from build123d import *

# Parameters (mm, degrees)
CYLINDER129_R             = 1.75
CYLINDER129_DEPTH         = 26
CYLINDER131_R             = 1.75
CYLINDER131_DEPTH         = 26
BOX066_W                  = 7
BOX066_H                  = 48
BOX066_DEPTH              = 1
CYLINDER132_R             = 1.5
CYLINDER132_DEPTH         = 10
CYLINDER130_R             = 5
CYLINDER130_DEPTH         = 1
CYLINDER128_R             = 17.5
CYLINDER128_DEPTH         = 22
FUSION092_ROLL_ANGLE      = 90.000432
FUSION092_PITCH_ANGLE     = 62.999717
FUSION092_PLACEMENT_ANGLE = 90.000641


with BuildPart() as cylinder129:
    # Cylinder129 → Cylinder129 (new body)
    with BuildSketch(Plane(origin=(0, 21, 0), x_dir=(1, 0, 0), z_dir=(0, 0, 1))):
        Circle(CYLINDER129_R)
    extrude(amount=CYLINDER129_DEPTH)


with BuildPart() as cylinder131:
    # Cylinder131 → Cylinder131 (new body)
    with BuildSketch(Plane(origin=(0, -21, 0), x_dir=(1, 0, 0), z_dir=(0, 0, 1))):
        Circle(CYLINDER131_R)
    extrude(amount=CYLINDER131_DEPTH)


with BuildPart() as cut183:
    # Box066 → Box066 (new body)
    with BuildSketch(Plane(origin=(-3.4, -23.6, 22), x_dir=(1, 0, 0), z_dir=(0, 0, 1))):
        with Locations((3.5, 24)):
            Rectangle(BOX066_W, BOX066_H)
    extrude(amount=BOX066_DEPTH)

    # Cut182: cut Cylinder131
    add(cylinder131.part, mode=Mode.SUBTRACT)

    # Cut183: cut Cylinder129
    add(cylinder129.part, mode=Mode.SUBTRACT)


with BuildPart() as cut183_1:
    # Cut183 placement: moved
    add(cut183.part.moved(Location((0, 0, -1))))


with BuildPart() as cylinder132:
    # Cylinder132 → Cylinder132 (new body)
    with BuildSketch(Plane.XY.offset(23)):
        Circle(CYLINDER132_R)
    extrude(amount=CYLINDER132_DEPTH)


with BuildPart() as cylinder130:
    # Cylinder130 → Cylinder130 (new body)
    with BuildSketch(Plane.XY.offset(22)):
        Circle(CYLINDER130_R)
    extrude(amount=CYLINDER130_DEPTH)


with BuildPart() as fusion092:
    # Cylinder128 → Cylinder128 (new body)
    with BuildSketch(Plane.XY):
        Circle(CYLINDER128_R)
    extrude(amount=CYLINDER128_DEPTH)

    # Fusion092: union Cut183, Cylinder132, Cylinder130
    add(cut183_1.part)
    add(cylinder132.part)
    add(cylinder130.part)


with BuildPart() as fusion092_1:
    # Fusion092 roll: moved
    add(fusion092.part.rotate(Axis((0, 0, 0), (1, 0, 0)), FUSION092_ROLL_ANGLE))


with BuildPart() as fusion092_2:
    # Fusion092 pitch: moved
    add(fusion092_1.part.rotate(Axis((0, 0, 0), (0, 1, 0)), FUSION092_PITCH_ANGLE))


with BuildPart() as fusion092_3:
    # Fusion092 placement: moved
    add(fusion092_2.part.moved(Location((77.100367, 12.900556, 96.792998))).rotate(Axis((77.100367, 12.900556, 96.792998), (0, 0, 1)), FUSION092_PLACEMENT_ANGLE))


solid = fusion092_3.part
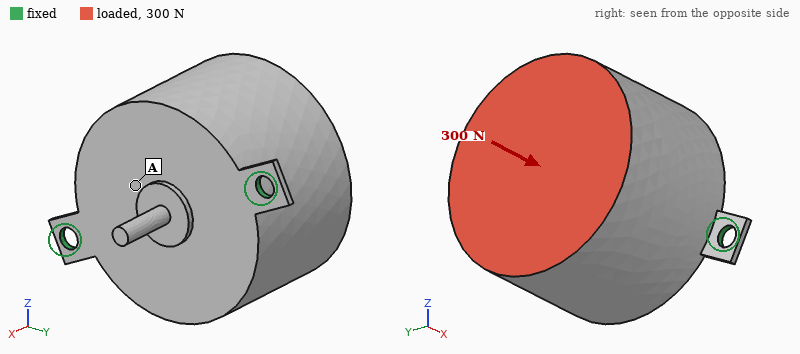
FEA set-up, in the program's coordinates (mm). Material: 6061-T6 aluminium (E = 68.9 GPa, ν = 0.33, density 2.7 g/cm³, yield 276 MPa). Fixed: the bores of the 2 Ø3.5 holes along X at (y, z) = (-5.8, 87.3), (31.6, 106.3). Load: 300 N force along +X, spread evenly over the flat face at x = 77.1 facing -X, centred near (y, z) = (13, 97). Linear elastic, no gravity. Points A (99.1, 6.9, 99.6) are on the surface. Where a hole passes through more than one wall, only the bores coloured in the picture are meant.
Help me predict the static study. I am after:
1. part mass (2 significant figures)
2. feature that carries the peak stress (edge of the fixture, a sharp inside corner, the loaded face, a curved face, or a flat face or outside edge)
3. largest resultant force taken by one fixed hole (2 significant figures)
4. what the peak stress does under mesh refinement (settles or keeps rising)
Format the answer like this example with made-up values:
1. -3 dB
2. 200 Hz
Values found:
1. 58 g
2. edge of the fixture
3. 170 N
4. keeps rising
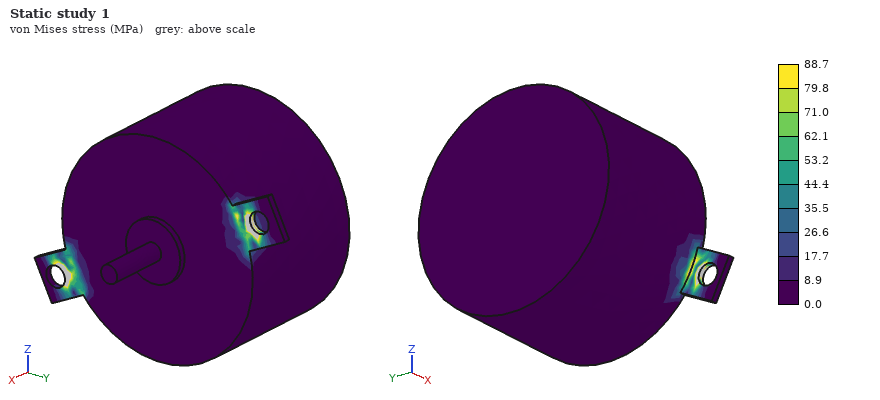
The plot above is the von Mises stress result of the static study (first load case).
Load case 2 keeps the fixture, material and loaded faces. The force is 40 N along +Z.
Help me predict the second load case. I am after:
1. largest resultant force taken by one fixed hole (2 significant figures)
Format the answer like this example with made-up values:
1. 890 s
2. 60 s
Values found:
1. 23 N
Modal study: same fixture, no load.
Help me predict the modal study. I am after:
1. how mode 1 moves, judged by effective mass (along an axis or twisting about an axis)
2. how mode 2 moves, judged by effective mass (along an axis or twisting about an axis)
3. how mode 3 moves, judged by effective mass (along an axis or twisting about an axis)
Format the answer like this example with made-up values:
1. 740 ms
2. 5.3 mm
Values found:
1. along Z
2. along X
3. along Y
